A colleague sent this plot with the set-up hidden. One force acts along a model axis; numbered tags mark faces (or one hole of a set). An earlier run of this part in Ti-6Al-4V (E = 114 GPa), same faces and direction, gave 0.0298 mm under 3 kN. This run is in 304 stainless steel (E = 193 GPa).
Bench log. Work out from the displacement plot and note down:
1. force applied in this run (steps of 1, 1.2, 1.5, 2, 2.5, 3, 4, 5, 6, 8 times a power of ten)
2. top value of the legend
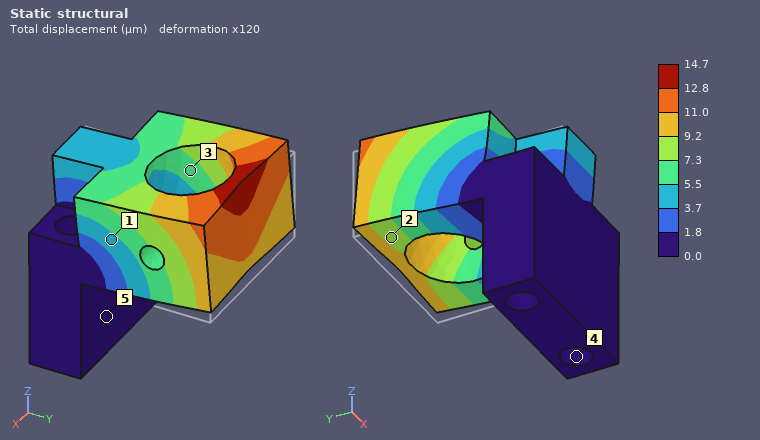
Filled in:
2.5 kN
14.7 µm
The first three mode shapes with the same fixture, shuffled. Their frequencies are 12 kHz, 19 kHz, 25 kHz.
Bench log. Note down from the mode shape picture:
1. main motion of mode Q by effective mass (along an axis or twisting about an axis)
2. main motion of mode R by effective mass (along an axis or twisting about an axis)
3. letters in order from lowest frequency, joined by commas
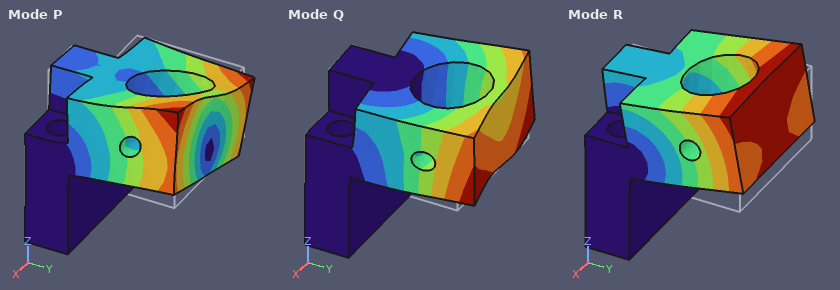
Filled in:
along X
along Z
R, Q, P
